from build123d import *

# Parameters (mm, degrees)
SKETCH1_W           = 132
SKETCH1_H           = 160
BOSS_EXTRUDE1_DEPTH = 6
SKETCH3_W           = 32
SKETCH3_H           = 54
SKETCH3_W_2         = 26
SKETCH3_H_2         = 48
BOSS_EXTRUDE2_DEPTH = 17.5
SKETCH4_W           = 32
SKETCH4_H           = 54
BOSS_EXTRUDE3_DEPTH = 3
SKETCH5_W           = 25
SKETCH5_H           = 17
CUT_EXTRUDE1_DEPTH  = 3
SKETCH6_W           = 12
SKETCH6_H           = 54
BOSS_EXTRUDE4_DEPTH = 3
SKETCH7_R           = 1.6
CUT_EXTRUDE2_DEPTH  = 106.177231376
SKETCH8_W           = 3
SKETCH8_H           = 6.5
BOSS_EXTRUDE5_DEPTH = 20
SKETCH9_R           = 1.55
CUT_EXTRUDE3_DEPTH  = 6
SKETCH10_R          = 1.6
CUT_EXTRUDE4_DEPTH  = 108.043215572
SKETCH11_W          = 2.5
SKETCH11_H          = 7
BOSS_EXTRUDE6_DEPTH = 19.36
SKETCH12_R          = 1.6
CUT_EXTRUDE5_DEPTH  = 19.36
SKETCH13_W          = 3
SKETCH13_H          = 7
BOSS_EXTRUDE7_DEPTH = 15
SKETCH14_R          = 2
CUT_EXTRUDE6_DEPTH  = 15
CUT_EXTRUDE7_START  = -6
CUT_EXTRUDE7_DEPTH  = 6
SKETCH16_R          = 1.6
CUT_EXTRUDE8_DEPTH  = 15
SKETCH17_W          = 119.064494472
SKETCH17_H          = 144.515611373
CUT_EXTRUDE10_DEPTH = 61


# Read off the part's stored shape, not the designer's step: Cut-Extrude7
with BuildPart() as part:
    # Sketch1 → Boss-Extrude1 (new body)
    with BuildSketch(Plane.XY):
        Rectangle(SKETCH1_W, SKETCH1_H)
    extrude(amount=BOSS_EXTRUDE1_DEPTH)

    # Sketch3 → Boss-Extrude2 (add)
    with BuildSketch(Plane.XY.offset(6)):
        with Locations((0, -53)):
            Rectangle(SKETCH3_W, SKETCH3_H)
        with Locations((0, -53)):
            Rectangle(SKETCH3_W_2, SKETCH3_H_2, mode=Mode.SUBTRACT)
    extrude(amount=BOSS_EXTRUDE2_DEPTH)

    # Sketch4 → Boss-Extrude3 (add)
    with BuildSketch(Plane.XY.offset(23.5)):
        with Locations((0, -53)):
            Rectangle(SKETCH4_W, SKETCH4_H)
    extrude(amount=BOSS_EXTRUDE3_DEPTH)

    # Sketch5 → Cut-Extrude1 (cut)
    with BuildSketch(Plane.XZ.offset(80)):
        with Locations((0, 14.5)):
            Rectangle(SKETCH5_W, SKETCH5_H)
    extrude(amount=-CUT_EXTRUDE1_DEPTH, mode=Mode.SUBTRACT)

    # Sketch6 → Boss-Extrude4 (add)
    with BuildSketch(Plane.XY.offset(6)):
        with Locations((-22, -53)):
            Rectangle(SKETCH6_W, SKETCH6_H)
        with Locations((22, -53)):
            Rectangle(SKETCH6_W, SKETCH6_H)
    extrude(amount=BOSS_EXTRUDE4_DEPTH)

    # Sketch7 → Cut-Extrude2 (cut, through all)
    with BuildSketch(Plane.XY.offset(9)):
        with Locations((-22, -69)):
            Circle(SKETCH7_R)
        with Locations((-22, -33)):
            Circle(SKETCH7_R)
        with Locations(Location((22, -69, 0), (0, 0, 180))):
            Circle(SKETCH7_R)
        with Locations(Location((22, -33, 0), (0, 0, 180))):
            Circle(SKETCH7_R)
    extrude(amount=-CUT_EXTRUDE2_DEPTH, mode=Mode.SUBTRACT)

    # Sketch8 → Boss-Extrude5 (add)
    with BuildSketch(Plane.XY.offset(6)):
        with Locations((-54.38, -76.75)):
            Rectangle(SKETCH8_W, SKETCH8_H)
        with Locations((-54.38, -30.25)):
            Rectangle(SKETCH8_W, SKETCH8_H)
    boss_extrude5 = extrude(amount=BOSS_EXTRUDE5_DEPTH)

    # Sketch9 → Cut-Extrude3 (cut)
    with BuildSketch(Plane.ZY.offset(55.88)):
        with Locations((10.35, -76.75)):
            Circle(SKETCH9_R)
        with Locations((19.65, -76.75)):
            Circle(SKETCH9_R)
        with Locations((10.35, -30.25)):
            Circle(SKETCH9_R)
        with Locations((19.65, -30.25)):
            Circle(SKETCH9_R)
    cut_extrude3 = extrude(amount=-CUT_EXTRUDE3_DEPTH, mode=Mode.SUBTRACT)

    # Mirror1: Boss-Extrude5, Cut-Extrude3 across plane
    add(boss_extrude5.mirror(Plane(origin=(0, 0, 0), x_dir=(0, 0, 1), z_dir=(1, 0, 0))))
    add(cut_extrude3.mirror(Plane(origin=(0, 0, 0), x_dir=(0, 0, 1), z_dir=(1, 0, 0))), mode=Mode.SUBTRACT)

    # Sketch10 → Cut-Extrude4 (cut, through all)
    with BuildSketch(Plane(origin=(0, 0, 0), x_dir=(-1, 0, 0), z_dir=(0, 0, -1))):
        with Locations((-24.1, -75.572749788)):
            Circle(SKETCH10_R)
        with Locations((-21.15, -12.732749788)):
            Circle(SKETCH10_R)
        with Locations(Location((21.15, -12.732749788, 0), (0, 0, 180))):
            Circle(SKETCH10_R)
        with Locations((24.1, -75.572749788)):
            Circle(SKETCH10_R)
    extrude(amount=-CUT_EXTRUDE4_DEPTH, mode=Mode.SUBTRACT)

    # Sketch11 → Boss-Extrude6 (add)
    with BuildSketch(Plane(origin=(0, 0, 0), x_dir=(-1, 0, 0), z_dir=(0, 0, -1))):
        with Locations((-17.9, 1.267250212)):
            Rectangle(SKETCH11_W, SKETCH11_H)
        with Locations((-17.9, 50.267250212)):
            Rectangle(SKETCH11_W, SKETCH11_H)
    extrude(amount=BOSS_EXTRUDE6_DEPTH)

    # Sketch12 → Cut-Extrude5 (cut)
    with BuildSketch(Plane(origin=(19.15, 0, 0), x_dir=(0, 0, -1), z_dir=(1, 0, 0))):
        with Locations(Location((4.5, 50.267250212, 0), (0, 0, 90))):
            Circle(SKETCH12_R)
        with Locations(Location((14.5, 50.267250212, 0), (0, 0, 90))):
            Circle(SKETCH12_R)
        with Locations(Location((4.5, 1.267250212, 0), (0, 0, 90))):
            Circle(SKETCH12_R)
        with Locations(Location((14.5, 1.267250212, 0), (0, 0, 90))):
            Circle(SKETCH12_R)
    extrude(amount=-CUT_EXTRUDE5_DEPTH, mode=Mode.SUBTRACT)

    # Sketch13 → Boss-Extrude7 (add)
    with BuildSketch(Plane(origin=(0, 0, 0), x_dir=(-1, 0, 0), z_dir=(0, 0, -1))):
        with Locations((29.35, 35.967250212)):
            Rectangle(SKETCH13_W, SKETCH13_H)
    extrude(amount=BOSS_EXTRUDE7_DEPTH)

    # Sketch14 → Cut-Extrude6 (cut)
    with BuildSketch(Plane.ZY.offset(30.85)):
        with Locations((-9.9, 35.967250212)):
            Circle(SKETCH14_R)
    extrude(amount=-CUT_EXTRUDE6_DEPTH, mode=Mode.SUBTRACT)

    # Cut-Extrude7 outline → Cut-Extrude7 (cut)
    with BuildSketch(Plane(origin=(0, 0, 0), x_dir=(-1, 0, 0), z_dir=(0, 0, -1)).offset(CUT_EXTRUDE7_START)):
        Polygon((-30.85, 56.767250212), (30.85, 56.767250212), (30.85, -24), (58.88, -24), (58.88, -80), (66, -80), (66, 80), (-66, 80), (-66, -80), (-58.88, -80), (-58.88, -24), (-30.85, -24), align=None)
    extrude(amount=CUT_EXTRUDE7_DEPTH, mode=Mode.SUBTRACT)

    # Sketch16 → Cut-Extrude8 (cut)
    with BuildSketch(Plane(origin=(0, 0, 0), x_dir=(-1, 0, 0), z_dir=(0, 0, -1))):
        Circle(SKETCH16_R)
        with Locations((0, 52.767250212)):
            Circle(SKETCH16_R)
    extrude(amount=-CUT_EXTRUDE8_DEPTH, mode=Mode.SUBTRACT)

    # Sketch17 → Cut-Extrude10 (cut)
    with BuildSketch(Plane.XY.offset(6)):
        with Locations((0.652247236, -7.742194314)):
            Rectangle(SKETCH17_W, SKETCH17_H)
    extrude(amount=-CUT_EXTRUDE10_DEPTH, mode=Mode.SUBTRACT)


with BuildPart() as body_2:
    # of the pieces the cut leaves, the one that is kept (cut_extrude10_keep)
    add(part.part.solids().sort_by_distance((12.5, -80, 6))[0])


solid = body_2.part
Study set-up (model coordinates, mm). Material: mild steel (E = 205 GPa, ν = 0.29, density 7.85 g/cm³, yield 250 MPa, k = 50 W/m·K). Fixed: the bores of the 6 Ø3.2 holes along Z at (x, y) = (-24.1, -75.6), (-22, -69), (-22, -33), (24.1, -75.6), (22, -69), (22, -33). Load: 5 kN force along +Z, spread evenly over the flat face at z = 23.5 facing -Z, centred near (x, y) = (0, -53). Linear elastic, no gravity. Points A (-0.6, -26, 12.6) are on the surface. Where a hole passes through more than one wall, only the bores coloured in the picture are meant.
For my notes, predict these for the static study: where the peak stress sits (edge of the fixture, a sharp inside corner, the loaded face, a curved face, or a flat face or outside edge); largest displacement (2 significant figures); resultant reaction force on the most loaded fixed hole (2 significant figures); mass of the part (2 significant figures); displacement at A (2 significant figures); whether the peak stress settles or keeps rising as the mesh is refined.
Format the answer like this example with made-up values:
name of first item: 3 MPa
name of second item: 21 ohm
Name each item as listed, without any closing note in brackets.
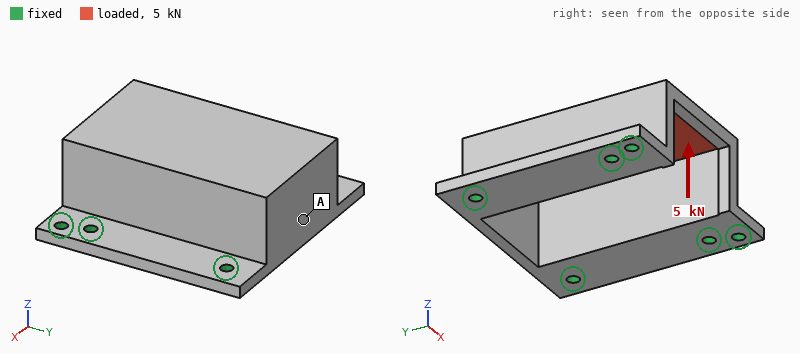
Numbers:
where the peak stress sits: edge of the fixture
largest displacement: 34 µm
resultant reaction force on the most loaded fixed hole: 1.3 kN
mass of the part: 130 g
displacement at A: 12 µm
whether the peak stress settles or keeps rising as the mesh is refined: keeps rising
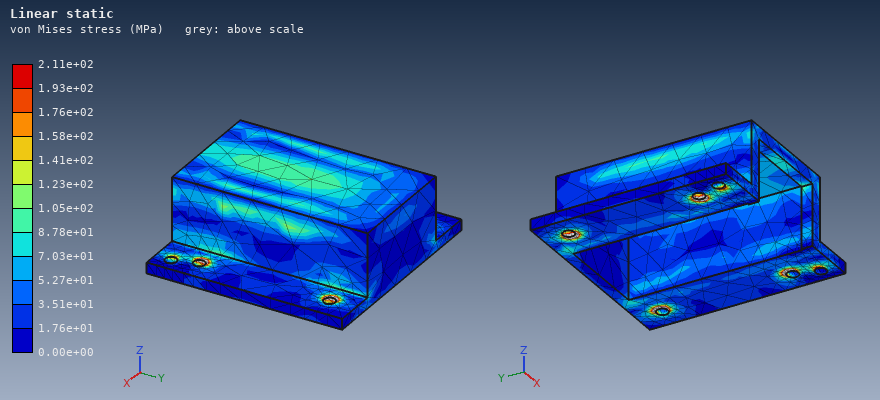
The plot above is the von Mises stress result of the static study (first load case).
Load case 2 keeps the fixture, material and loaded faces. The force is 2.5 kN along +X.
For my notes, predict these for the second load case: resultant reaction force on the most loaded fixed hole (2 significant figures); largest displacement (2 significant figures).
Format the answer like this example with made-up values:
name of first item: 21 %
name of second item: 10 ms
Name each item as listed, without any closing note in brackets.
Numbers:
resultant reaction force on the most loaded fixed hole: 1.3 kN
largest displacement: 45 µm
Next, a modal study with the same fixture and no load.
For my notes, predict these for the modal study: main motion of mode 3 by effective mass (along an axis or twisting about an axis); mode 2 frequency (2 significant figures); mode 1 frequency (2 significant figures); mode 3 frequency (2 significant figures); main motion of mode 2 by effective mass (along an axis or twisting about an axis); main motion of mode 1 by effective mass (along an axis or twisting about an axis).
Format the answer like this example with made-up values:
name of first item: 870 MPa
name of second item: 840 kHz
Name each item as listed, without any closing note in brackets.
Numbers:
main motion of mode 3 by effective mass: along Z
mode 2 frequency: 8600 Hz
mode 1 frequency: 5700 Hz
mode 3 frequency: 9900 Hz
main motion of mode 2 by effective mass: along Y
main motion of mode 1 by effective mass: along X
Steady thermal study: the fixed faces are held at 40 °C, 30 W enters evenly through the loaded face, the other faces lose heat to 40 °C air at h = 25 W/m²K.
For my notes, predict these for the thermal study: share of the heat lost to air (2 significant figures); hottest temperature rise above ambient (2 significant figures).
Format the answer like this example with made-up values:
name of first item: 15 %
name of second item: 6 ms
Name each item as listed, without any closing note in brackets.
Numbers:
share of the heat lost to air: 21 %
hottest temperature rise above ambient: 54 K
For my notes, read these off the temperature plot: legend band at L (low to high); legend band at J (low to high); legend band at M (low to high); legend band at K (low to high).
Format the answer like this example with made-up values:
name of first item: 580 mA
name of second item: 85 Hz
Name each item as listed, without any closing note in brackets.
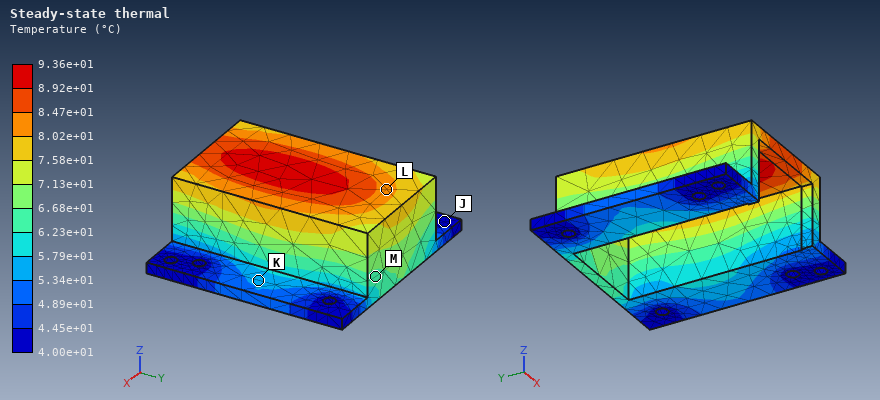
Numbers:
legend band at L: 8.02e+01 to 8.47e+01 °C
legend band at J: 4.00e+01 to 4.45e+01 °C
legend band at M: 6.23e+01 to 6.68e+01 °C
legend band at K: 5.34e+01 to 5.79e+01 °C
